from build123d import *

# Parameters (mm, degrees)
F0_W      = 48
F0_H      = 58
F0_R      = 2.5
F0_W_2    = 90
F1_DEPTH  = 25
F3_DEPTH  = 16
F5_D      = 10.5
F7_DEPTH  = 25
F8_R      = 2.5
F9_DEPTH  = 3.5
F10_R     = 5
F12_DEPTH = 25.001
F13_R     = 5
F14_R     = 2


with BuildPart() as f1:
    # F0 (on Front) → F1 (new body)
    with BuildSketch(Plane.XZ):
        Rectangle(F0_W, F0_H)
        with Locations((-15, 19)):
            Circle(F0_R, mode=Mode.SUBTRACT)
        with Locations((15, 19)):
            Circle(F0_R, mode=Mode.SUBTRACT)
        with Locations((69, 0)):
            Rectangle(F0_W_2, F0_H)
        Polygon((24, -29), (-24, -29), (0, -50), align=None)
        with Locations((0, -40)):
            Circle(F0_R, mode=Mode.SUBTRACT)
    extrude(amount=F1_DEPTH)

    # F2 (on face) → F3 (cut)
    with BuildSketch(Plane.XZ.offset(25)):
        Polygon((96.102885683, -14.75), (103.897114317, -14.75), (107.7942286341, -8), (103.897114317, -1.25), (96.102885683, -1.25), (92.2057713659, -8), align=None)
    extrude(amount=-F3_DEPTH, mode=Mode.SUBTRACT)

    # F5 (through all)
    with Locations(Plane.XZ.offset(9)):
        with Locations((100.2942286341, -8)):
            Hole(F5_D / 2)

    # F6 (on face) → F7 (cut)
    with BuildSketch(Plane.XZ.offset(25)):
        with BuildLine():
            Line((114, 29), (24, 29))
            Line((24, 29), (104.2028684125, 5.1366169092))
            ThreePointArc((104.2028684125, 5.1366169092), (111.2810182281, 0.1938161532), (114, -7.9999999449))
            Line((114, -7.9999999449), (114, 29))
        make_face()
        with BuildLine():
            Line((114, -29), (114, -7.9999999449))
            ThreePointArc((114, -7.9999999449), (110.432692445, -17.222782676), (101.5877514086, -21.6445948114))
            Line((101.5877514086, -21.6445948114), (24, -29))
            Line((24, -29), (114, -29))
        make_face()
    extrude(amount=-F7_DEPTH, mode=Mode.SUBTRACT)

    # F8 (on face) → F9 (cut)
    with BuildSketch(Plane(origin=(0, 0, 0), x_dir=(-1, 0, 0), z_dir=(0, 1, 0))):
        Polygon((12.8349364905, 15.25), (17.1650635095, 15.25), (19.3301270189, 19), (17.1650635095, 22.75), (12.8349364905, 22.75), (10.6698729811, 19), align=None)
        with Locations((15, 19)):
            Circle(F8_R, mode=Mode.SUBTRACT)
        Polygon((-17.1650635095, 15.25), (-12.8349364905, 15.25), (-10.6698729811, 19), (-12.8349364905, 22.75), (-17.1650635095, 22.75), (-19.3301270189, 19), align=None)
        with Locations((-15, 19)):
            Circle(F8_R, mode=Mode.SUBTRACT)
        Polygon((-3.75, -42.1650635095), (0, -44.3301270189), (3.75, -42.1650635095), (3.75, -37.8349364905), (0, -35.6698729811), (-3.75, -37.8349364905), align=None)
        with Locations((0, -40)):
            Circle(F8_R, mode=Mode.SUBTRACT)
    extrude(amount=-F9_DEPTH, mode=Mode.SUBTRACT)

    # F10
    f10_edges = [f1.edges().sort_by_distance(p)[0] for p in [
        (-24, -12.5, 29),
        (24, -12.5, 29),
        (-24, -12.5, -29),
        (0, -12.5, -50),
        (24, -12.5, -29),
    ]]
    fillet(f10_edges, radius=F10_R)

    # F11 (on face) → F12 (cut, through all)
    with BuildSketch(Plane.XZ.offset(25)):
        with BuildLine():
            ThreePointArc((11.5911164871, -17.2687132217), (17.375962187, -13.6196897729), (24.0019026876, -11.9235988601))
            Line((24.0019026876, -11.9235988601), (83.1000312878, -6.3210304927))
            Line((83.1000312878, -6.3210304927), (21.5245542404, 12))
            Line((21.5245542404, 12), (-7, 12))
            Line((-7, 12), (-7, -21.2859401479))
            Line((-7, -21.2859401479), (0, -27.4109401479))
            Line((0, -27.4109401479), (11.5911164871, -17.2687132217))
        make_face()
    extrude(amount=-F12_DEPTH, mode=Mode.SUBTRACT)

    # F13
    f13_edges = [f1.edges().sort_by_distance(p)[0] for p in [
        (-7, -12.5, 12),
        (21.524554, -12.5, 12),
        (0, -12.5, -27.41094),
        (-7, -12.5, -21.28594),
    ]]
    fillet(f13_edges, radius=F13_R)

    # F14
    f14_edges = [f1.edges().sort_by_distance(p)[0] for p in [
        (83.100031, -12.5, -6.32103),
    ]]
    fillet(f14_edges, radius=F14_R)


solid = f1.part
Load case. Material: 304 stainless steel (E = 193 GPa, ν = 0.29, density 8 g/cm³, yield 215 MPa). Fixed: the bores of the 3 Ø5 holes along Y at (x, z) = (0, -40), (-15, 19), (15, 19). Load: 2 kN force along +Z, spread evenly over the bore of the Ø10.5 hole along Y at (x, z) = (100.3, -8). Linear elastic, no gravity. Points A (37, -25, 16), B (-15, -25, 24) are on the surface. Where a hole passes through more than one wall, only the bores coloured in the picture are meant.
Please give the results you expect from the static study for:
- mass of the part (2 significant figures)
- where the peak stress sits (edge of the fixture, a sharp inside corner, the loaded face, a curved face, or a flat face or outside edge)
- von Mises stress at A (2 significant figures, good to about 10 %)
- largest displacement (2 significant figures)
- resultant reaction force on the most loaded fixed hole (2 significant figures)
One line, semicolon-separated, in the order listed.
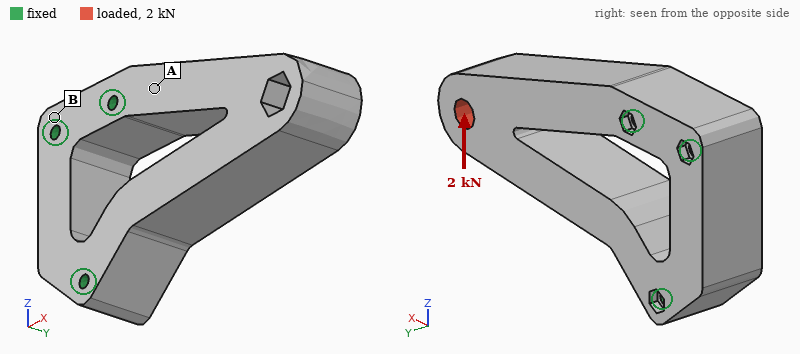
1.0 kg; edge of the fixture; 7.7 MPa; 22 µm; 3.0 kN
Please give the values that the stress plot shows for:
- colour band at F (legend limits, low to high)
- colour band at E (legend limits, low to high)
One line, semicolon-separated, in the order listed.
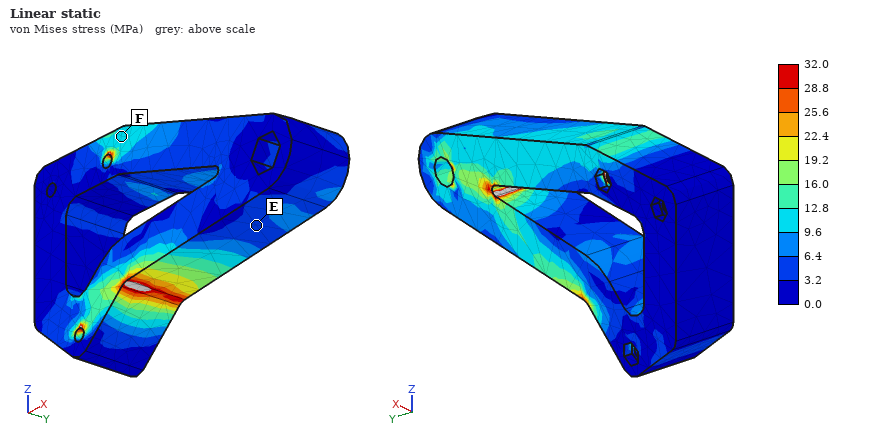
9.6 to 12.8 MPa; 3.2 to 6.4 MPa
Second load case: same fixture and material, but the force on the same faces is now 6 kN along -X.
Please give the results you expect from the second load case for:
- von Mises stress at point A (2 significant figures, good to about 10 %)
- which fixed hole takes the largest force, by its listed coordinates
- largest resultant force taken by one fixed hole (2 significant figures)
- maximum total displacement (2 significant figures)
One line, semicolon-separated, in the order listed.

11 MPa; (0, -40); 3.3 kN; 41 µm
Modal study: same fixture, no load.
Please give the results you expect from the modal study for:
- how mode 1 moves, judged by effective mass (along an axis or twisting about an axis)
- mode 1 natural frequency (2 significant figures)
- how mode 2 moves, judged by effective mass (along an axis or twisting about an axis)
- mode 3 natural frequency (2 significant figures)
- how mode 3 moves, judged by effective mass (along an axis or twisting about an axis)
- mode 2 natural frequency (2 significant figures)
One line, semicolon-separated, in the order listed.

along Y; 1700 Hz; along Z; 5700 Hz; along X; 3600 Hz
